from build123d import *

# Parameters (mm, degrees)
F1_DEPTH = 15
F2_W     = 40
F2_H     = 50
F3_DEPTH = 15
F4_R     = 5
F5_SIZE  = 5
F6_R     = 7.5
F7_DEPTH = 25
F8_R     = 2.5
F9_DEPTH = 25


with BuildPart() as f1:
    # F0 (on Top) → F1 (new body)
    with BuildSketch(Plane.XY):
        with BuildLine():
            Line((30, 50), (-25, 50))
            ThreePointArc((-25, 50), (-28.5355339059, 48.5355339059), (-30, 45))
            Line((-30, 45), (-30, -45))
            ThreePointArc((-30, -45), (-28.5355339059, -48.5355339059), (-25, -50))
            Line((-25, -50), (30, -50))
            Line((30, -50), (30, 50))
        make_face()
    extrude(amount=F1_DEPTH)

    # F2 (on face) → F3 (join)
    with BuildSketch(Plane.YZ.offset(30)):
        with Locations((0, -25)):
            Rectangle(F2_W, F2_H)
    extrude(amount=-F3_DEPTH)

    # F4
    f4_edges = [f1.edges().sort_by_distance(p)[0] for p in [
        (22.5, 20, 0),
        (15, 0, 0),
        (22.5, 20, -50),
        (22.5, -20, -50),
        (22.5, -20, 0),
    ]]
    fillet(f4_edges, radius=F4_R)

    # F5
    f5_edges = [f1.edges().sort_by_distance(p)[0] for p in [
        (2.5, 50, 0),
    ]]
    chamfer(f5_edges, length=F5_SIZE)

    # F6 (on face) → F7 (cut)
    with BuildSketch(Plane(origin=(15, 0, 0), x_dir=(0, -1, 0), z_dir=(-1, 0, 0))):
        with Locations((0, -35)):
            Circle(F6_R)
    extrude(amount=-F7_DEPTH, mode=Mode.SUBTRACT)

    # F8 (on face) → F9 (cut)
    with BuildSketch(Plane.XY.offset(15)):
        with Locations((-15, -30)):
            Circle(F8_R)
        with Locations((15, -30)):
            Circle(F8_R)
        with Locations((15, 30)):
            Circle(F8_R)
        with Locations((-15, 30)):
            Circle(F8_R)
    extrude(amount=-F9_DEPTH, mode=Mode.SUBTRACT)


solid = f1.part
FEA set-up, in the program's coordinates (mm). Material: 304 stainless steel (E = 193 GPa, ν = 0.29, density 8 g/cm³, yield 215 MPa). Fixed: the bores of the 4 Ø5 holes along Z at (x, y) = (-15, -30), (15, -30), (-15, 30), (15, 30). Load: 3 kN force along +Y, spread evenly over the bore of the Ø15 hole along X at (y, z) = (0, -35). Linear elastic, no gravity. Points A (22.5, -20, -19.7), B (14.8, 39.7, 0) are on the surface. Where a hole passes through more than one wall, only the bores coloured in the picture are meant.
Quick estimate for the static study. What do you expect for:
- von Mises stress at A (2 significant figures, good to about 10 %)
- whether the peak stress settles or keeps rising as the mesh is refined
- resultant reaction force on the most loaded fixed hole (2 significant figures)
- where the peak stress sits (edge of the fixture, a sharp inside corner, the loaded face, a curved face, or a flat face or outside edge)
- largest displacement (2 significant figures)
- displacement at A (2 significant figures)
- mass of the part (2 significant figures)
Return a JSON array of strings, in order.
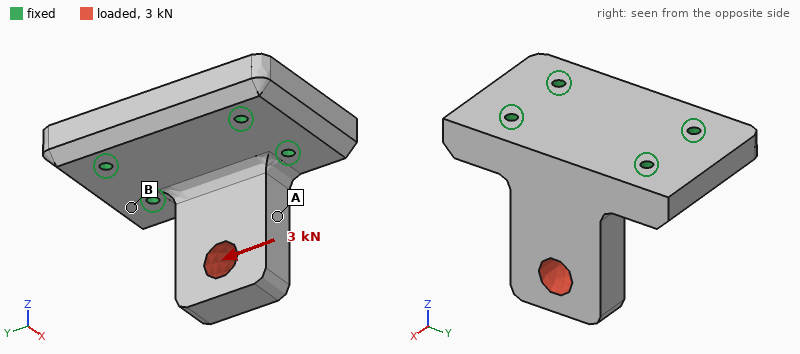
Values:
["14 MPa", "keeps rising", "2.7 kN", "a sharp inside corner", "15 µm", "6.7 µm", "910 g"]
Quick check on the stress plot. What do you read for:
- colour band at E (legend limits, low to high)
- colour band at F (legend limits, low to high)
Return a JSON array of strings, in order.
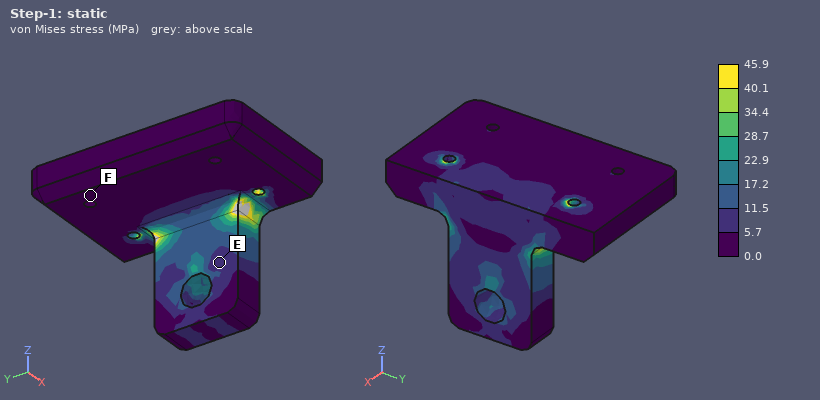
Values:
["5.7 to 11.5 MPa", "0.0 to 5.7 MPa"]
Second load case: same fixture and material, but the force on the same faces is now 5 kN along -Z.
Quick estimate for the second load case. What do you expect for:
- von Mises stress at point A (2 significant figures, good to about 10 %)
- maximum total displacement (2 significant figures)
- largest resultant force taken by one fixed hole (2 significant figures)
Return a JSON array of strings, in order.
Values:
["8.3 MPa", "12 µm", "2.8 kN"]
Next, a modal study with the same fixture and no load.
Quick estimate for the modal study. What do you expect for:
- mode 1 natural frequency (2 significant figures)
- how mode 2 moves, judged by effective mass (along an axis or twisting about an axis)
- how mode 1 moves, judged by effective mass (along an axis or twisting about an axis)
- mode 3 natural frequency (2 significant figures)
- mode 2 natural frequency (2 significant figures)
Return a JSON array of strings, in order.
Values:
["3400 Hz", "along Y", "along X", "9300 Hz", "7000 Hz"]
